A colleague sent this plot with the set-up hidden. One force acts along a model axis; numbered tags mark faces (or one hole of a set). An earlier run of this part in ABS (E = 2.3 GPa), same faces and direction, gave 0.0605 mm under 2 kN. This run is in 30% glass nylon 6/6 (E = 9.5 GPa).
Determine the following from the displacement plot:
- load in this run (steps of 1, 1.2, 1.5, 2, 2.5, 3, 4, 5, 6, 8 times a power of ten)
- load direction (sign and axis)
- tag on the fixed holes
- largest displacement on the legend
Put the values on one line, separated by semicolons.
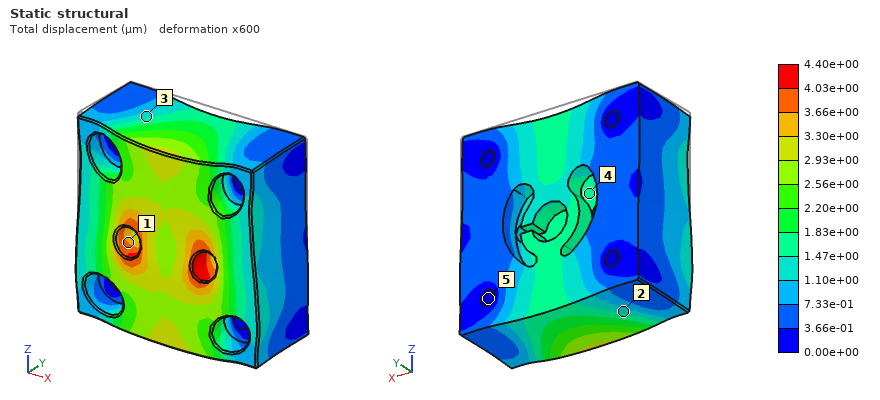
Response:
600 N; -Z; 5; 4.40e+00 µm
